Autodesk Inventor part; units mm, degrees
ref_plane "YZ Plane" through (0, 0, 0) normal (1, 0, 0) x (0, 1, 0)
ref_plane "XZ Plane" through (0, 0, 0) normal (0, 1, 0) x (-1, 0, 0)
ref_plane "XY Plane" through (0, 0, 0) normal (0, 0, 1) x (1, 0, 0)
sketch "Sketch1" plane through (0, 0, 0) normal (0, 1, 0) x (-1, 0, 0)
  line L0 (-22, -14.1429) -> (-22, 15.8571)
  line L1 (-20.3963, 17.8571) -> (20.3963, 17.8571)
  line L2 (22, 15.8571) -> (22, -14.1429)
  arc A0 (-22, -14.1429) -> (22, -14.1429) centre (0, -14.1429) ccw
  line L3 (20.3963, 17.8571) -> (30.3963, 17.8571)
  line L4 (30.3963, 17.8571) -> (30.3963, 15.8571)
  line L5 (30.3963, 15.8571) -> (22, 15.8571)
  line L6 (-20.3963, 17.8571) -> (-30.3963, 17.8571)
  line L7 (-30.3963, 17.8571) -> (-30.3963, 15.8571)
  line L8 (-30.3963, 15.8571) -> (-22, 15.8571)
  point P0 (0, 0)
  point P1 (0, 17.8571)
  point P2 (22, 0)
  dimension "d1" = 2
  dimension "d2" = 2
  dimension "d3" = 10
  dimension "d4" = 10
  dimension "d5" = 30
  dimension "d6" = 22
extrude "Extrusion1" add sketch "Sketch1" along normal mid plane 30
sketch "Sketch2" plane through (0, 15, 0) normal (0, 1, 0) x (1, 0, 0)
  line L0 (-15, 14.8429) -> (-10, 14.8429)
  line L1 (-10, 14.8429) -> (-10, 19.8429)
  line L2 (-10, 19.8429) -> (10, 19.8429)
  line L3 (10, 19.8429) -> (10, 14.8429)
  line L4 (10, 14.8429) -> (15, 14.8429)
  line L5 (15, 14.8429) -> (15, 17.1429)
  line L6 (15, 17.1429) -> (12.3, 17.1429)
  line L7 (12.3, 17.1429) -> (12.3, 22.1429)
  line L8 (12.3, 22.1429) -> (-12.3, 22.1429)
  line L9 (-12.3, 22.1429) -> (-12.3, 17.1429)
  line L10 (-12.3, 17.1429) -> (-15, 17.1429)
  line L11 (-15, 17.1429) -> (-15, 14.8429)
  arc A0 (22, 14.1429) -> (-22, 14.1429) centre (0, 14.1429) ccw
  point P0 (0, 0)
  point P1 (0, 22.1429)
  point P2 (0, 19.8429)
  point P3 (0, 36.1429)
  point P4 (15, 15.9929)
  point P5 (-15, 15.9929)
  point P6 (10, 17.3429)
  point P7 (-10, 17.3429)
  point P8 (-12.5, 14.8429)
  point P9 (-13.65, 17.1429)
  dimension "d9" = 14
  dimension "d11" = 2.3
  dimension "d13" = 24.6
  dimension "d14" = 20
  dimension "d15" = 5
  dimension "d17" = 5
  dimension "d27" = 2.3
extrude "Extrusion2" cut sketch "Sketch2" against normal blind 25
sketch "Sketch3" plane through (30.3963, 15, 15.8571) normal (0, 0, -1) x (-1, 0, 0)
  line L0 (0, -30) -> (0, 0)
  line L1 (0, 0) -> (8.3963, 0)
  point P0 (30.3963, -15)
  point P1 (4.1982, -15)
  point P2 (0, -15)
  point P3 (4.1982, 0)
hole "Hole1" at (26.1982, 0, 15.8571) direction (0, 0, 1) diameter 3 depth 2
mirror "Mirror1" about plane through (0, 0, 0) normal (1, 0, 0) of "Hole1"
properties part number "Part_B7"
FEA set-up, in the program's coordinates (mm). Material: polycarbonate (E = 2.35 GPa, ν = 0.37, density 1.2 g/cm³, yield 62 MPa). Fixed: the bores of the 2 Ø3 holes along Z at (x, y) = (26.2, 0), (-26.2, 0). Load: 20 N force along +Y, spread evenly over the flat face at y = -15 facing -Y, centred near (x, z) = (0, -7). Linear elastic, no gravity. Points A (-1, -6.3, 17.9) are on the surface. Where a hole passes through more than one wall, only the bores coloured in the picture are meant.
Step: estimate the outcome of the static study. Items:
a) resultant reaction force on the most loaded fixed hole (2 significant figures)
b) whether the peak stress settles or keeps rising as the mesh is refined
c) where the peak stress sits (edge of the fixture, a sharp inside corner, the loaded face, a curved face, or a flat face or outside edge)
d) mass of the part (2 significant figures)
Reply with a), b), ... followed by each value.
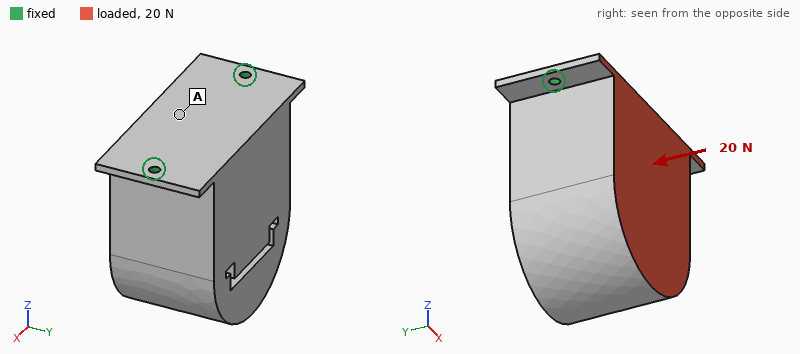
a) 10 N
b) keeps rising
c) edge of the fixture
d) 76 g
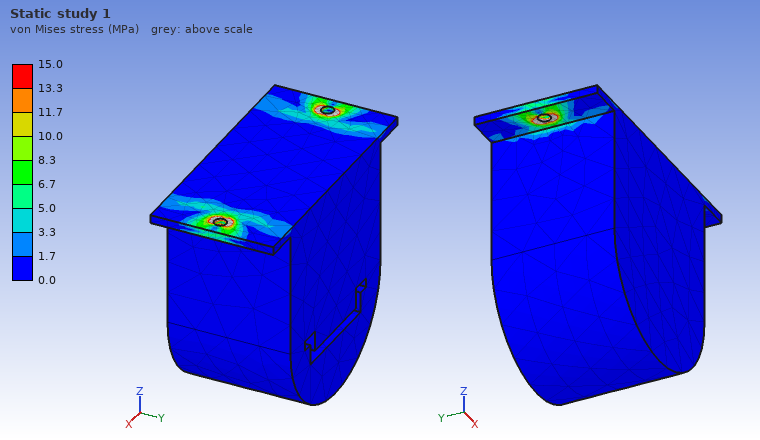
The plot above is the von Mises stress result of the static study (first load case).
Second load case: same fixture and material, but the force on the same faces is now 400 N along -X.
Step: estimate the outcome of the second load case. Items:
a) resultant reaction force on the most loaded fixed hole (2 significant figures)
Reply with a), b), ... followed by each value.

a) 300 N
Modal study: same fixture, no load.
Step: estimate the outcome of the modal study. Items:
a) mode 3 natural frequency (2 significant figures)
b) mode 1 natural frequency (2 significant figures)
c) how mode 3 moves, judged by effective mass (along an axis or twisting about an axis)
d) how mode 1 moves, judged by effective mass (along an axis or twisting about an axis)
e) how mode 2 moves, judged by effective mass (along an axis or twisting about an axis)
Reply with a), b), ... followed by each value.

a) 920 Hz
b) 100 Hz
c) along Z
d) along Y
e) along X
